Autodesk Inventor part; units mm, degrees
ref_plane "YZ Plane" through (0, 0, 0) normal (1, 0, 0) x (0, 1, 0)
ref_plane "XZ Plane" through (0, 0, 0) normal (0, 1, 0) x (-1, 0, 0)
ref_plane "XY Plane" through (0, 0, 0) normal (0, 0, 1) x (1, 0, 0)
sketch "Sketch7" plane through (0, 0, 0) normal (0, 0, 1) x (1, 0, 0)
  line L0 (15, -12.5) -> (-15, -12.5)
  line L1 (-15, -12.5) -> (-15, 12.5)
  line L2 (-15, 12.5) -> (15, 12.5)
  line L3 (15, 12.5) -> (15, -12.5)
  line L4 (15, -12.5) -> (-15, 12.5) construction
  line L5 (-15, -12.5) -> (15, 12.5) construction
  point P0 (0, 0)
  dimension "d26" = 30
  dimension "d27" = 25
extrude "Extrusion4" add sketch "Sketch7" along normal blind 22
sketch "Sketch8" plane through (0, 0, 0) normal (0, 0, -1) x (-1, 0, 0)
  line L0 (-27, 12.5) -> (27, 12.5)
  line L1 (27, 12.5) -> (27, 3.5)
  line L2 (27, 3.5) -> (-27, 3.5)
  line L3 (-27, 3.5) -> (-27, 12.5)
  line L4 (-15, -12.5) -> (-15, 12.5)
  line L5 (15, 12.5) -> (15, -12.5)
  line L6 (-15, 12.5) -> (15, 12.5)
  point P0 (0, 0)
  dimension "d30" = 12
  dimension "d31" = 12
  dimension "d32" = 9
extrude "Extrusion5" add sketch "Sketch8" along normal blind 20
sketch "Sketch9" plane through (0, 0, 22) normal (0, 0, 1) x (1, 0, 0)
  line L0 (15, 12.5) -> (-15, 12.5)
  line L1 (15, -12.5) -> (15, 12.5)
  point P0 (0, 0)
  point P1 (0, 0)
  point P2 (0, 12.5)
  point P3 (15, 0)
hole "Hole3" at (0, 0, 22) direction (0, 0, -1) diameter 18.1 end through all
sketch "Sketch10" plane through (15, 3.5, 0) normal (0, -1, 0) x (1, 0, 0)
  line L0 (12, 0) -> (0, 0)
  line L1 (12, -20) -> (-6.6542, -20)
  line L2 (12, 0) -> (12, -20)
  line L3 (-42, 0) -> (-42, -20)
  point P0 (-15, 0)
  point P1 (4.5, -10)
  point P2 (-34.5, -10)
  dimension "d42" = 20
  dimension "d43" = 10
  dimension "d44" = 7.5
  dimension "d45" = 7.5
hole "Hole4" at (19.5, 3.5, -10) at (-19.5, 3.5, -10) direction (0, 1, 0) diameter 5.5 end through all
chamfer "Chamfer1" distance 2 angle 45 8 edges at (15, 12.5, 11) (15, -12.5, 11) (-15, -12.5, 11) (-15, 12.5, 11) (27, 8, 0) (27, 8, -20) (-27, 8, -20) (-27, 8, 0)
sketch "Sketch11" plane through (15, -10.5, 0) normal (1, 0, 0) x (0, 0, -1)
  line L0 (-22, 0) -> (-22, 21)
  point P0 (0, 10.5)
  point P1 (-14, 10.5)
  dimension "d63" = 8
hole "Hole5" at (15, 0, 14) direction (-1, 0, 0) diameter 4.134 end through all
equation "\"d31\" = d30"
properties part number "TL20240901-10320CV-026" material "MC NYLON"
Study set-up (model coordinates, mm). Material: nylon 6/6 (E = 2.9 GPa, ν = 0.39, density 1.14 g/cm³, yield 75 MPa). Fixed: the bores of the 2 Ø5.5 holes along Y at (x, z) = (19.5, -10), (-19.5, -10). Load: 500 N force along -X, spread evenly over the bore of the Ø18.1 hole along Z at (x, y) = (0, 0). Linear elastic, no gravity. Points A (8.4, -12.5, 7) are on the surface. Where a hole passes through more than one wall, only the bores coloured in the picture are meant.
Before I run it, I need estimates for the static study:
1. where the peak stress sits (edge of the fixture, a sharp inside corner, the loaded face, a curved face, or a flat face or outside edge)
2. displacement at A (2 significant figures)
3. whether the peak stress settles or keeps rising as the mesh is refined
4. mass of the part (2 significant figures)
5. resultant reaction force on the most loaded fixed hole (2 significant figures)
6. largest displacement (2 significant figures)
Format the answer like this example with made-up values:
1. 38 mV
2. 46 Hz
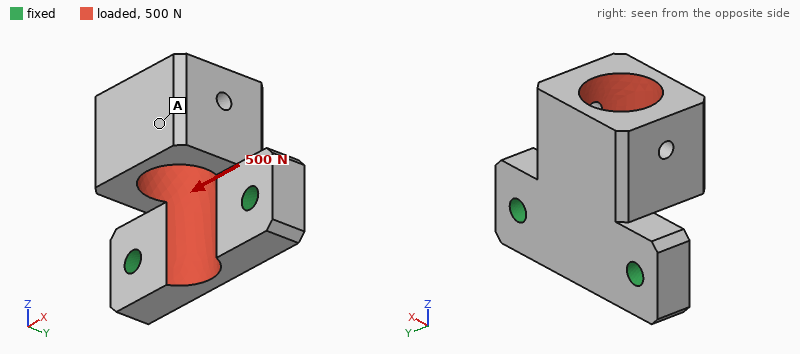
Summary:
1. a sharp inside corner
2. 0.13 mm
3. keeps rising
4. 21 g
5. 320 N
6. 0.14 mm
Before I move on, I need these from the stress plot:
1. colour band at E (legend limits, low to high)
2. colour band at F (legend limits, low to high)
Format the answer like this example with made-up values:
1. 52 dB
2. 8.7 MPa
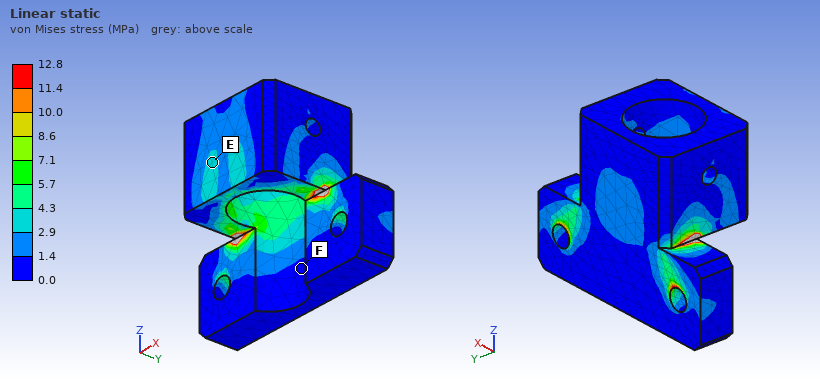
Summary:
1. 2.9 to 4.3 MPa
2. 0.0 to 1.4 MPa
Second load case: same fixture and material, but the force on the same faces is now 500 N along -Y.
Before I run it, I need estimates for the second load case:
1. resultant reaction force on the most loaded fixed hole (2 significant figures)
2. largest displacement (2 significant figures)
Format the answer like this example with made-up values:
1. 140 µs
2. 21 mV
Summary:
1. 250 N
2. 0.74 mm
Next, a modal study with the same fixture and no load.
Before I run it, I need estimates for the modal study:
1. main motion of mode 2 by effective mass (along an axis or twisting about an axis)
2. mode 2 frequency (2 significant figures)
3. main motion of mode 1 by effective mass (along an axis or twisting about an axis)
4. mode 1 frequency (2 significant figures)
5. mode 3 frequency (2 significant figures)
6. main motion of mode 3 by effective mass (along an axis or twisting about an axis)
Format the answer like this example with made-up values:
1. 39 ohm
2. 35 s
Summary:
1. along X
2. 2500 Hz
3. along Y
4. 1100 Hz
5. 4100 Hz
6. along X
